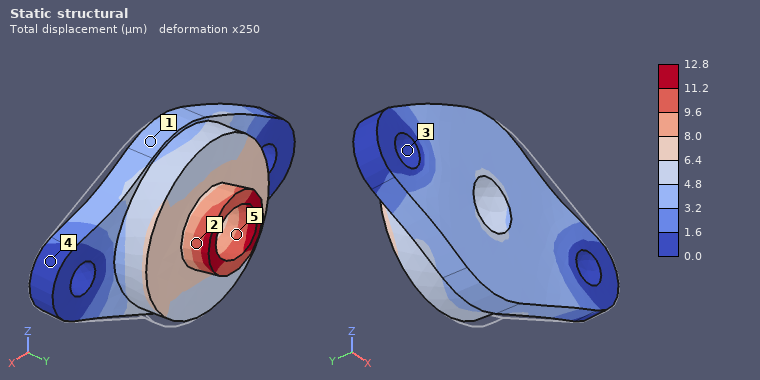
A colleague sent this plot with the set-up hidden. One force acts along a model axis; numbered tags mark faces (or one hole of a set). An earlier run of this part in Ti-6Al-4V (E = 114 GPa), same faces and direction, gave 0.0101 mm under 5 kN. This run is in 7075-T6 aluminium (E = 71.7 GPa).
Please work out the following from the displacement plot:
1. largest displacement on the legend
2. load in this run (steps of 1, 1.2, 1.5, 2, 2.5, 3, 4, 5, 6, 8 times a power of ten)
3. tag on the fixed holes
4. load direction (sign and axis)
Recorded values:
12.8 µm
4 kN
3
-X
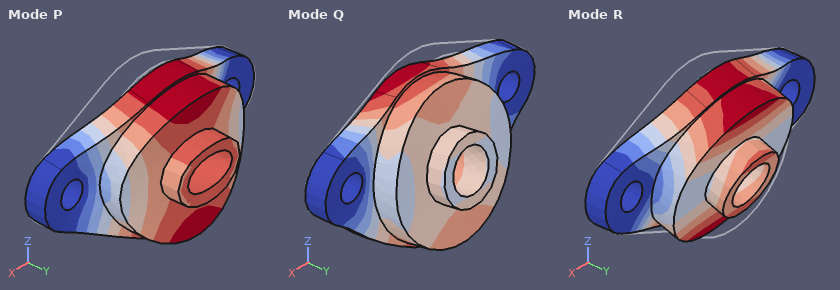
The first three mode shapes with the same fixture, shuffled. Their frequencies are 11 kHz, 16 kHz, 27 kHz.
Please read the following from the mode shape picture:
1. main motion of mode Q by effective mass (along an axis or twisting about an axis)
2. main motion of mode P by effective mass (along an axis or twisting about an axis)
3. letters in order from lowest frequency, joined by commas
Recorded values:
along Z
along Y
R, P, Q
